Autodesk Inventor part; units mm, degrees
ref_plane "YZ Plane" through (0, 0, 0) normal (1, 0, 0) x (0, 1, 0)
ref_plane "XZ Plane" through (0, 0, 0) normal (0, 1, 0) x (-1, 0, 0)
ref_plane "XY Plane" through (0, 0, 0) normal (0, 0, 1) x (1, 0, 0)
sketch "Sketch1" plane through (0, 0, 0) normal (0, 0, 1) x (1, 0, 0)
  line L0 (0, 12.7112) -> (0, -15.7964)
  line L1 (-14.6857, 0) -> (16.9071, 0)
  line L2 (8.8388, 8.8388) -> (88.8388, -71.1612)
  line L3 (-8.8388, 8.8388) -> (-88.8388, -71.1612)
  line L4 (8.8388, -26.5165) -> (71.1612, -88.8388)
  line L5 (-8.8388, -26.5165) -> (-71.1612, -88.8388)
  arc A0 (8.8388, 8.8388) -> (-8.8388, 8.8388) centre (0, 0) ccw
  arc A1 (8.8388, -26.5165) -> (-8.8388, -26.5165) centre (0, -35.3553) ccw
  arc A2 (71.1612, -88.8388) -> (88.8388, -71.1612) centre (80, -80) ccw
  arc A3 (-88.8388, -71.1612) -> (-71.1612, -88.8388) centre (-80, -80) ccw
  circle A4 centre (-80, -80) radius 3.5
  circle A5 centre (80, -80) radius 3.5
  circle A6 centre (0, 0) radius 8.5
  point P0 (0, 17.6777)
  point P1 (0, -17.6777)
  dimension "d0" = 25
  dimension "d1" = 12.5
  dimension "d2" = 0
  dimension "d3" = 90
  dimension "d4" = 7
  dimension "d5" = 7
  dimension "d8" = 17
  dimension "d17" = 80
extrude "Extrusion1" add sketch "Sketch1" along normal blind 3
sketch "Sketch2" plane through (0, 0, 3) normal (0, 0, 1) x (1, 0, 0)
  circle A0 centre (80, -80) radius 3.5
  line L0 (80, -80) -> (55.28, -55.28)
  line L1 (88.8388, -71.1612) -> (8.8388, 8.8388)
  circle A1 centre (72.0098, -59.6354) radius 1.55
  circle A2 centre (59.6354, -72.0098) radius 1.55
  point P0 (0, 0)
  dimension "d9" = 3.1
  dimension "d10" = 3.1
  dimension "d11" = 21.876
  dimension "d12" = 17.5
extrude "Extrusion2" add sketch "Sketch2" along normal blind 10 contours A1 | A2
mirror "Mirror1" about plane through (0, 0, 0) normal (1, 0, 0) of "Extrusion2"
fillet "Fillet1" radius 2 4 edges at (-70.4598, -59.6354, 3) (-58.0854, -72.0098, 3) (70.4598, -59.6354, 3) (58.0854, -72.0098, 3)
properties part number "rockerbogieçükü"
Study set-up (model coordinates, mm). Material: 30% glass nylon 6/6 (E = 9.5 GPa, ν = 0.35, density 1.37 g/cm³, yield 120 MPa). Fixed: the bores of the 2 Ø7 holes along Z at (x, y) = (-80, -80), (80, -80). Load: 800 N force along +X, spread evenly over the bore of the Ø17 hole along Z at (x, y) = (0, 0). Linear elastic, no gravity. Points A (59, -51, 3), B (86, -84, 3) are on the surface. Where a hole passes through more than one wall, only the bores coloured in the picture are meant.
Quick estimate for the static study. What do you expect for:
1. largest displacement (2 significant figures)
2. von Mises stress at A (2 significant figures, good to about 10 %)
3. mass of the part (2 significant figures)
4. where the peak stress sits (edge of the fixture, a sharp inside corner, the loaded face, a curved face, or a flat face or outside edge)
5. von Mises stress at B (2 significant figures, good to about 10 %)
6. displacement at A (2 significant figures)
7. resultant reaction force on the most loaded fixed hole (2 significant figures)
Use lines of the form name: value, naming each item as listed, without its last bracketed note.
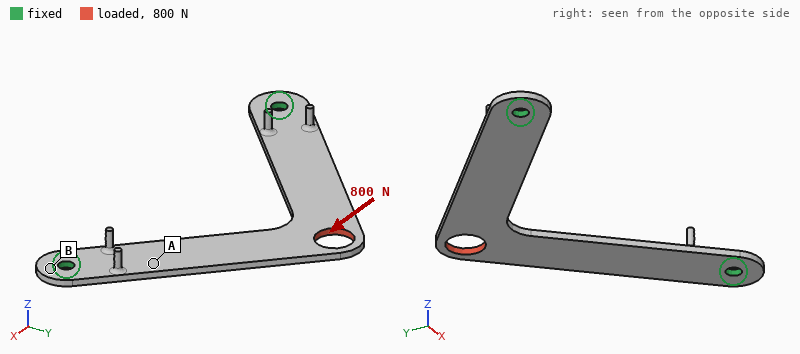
largest displacement: 0.21 mm
von Mises stress at A: 8.1 MPa
mass of the part: 24 g
where the peak stress sits: the loaded face
von Mises stress at B: 3.3 MPa
displacement at A: 0.041 mm
resultant reaction force on the most loaded fixed hole: 560 N
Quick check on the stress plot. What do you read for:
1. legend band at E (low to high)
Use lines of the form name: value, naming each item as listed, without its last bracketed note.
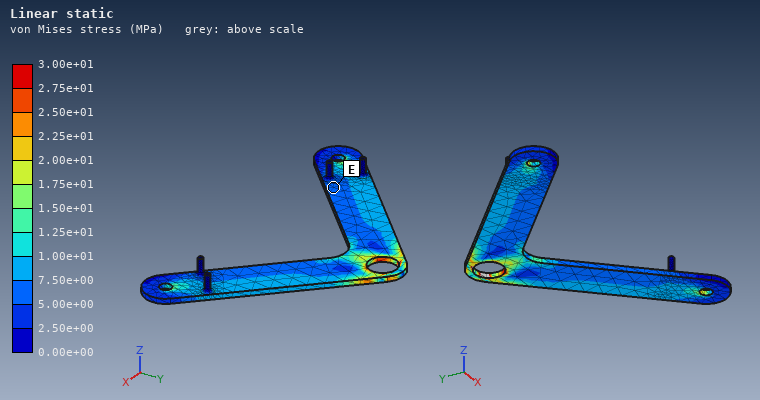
legend band at E: 5.00e+00 to 7.50e+00 MPa
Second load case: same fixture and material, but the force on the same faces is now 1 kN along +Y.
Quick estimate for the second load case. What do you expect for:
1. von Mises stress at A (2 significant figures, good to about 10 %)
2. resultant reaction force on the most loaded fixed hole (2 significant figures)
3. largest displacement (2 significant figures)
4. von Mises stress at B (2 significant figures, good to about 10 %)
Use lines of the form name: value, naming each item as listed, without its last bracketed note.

von Mises stress at A: 8.7 MPa
resultant reaction force on the most loaded fixed hole: 690 N
largest displacement: 0.18 mm
von Mises stress at B: 3.8 MPa
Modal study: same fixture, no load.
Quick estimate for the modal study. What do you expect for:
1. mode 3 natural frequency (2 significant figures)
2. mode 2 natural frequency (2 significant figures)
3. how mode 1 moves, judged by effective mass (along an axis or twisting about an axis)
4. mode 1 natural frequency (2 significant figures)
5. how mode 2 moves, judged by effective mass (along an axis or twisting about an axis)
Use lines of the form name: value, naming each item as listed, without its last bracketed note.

mode 3 natural frequency: 690 Hz
mode 2 natural frequency: 490 Hz
how mode 1 moves, judged by effective mass: along Z
mode 1 natural frequency: 140 Hz
how mode 2 moves, judged by effective mass: twisting about Y
